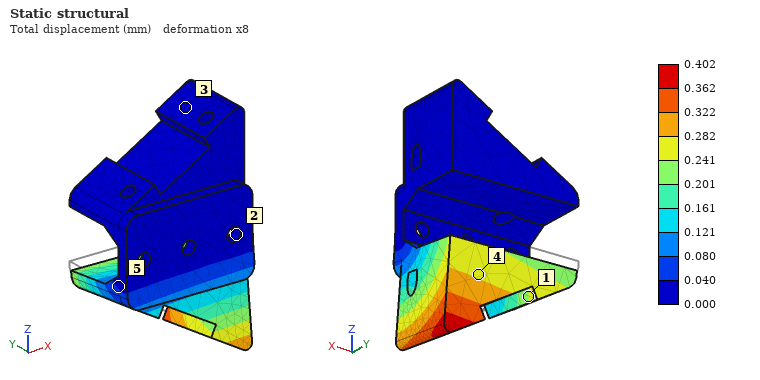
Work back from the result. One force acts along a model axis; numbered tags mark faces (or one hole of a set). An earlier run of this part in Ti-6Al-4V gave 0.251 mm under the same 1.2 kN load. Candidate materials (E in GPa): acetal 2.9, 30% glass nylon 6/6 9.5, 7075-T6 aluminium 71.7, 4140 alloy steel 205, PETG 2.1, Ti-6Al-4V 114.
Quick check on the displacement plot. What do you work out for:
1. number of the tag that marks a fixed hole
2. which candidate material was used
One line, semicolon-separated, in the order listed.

2; 7075-T6 aluminium
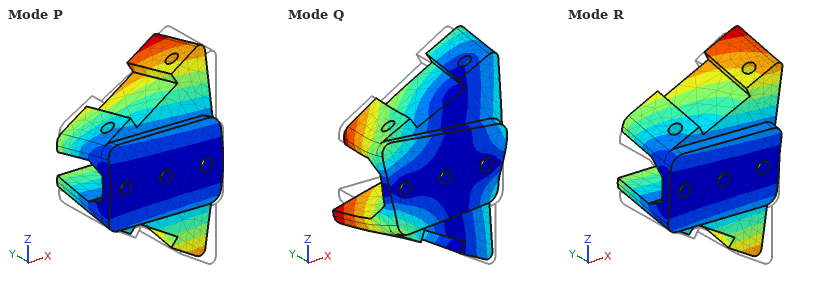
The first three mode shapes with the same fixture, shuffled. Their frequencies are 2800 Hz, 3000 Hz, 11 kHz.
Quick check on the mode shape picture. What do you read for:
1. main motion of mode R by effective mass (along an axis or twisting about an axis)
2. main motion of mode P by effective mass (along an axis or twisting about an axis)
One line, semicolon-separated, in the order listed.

along Z; along Y
